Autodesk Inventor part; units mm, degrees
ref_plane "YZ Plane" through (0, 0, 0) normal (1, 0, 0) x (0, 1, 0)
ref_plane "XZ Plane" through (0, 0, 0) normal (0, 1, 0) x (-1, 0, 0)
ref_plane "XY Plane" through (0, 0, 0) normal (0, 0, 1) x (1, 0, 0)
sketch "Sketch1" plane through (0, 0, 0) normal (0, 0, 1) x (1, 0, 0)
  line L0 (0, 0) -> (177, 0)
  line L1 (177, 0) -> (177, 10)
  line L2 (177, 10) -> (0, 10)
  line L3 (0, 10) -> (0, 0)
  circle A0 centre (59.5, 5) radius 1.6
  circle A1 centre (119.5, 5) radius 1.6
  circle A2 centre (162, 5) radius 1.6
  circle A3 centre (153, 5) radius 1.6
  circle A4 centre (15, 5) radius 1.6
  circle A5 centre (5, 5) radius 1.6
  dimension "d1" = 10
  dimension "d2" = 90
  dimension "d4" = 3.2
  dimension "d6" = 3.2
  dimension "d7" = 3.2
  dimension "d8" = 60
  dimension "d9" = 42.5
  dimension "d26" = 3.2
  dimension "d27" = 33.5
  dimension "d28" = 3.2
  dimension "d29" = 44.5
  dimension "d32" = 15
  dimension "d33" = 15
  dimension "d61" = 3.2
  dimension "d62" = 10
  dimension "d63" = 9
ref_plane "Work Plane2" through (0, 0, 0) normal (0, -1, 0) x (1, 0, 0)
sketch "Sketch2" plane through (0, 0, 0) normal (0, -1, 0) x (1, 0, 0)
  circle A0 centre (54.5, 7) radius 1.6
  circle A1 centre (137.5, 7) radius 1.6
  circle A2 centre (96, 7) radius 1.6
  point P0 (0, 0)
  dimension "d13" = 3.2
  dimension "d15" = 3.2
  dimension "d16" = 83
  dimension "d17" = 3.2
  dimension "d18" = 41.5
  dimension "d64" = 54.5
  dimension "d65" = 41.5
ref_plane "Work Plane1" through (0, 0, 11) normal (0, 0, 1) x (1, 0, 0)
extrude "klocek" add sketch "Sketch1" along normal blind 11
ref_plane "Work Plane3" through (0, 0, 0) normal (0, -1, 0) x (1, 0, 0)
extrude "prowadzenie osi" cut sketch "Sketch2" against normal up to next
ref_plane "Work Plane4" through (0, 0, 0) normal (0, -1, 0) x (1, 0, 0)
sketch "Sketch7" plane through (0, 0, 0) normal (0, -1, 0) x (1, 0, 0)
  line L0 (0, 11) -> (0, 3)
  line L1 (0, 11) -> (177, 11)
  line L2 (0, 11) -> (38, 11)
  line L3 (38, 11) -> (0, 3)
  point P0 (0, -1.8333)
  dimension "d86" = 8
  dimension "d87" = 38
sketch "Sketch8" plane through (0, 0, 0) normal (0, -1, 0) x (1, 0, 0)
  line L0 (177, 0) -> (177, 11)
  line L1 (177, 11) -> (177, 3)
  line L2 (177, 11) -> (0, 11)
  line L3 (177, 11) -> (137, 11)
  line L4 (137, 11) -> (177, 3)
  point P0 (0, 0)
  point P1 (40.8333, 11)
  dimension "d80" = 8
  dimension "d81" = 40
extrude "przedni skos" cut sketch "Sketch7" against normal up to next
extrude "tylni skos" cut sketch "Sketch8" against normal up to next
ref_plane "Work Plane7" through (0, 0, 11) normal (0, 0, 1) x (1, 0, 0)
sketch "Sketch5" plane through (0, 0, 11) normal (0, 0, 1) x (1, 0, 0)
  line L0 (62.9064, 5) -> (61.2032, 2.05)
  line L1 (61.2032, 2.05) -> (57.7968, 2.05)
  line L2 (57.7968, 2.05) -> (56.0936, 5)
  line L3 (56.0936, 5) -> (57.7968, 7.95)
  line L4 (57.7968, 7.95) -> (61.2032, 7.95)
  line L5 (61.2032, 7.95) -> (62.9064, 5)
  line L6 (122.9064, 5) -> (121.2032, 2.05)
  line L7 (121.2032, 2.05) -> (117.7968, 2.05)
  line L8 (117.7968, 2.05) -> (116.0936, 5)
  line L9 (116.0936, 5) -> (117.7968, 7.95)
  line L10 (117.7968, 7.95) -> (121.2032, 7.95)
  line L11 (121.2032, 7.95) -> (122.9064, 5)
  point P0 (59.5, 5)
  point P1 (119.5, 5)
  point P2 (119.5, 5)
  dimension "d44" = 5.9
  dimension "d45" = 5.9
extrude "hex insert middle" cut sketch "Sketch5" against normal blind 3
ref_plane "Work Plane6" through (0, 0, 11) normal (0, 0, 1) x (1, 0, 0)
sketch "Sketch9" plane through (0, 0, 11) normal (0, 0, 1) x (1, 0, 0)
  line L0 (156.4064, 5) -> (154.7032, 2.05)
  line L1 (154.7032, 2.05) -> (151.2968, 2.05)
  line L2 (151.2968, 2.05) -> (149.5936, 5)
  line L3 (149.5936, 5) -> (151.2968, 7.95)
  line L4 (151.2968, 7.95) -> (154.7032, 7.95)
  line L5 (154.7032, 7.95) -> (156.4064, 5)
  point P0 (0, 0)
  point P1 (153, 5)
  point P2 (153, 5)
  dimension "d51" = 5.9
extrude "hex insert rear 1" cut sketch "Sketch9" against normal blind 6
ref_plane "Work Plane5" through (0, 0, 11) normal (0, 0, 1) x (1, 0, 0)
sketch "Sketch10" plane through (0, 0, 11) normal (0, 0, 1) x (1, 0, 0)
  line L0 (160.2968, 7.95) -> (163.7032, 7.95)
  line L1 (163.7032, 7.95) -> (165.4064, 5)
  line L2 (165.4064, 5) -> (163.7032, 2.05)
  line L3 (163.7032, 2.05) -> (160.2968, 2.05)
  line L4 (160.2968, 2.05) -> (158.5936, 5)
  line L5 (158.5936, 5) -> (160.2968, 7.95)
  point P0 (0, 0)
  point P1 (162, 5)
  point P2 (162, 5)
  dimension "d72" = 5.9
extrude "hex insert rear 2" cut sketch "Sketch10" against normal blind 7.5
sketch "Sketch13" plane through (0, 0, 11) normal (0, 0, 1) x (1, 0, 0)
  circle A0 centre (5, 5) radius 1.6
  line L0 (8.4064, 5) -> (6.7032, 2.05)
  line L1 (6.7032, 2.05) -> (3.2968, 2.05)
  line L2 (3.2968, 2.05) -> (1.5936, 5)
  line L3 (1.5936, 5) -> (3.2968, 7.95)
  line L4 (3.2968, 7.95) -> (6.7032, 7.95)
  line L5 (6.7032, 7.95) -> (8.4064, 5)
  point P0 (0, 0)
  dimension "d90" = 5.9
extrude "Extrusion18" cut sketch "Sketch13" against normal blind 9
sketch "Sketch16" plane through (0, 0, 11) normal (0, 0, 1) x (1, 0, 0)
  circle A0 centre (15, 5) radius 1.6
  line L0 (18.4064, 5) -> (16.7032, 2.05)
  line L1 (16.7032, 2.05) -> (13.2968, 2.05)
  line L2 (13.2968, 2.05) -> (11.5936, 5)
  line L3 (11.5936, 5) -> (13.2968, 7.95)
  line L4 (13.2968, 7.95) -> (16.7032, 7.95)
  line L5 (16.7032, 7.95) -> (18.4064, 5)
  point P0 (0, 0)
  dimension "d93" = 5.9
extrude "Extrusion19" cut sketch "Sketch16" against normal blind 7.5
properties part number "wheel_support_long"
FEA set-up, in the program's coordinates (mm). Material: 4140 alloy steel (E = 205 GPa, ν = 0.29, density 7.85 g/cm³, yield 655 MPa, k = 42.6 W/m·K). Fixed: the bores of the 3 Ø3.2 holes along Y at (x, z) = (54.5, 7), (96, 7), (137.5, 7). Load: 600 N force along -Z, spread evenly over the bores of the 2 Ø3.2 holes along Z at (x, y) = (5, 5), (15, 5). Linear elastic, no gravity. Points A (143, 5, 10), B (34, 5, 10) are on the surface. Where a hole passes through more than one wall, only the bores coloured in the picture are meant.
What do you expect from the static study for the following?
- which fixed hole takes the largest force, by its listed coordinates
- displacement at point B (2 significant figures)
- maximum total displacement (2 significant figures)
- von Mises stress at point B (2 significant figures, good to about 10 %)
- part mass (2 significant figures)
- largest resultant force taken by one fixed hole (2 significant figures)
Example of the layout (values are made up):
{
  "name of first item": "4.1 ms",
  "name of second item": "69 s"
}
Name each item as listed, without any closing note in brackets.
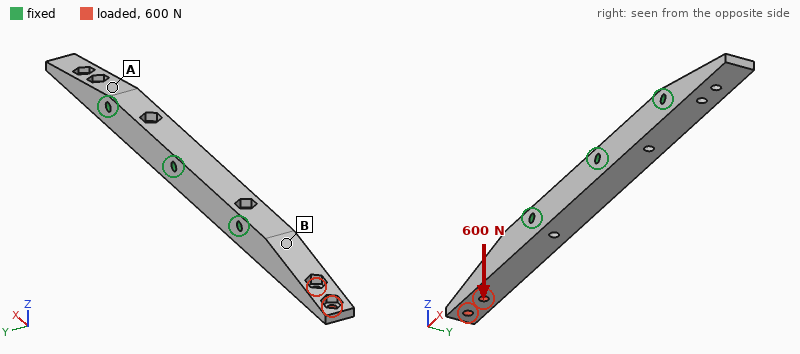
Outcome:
{
  "which fixed hole takes the largest force, by its listed coordinates": "(54.5, 7)",
  "displacement at point B": "0.035 mm",
  "maximum total displacement": "0.17 mm",
  "von Mises stress at point B": "82 MPa",
  "part mass": "120 g",
  "largest resultant force taken by one fixed hole": "1.1 kN"
}
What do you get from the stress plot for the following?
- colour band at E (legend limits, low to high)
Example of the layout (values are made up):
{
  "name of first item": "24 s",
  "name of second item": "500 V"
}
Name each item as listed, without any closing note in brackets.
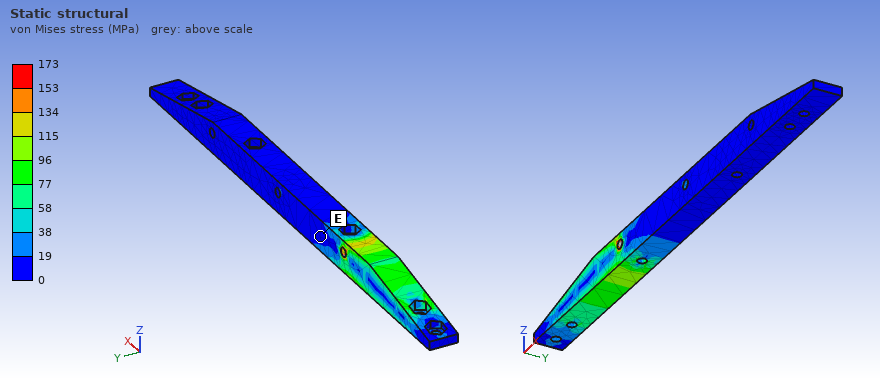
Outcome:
{
  "colour band at E": "0 to 19 MPa"
}
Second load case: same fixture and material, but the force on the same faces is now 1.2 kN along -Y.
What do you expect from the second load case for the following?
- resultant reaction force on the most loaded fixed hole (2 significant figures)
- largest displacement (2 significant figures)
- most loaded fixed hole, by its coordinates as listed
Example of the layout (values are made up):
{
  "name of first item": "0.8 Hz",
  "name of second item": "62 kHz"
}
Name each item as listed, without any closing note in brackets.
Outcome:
{
  "resultant reaction force on the most loaded fixed hole": "1.4 kN",
  "largest displacement": "0.28 mm",
  "most loaded fixed hole, by its coordinates as listed": "(54.5, 7)"
}
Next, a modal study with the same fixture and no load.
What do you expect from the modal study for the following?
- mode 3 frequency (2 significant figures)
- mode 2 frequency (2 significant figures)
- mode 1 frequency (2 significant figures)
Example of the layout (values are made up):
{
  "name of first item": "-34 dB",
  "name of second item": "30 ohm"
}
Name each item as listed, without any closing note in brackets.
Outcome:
{
  "mode 3 frequency": "5400 Hz",
  "mode 2 frequency": "4000 Hz",
  "mode 1 frequency": "3800 Hz"
}
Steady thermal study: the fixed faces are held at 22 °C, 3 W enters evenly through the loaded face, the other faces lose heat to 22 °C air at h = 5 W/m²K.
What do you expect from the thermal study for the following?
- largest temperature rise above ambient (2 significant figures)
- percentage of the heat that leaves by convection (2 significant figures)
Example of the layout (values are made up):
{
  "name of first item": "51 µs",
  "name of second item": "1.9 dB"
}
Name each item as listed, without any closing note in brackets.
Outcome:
{
  "largest temperature rise above ambient": "40 K",
  "percentage of the heat that leaves by convection": "6.3 %"
}
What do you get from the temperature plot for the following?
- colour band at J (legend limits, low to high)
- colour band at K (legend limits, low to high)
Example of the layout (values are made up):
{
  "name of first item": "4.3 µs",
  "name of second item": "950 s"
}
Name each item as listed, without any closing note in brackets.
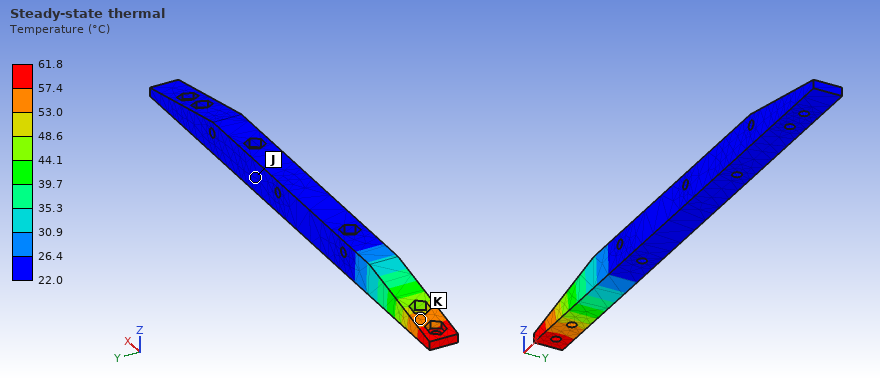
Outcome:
{
  "colour band at J": "22.0 to 26.4 °C",
  "colour band at K": "53.0 to 57.4 °C"
}
